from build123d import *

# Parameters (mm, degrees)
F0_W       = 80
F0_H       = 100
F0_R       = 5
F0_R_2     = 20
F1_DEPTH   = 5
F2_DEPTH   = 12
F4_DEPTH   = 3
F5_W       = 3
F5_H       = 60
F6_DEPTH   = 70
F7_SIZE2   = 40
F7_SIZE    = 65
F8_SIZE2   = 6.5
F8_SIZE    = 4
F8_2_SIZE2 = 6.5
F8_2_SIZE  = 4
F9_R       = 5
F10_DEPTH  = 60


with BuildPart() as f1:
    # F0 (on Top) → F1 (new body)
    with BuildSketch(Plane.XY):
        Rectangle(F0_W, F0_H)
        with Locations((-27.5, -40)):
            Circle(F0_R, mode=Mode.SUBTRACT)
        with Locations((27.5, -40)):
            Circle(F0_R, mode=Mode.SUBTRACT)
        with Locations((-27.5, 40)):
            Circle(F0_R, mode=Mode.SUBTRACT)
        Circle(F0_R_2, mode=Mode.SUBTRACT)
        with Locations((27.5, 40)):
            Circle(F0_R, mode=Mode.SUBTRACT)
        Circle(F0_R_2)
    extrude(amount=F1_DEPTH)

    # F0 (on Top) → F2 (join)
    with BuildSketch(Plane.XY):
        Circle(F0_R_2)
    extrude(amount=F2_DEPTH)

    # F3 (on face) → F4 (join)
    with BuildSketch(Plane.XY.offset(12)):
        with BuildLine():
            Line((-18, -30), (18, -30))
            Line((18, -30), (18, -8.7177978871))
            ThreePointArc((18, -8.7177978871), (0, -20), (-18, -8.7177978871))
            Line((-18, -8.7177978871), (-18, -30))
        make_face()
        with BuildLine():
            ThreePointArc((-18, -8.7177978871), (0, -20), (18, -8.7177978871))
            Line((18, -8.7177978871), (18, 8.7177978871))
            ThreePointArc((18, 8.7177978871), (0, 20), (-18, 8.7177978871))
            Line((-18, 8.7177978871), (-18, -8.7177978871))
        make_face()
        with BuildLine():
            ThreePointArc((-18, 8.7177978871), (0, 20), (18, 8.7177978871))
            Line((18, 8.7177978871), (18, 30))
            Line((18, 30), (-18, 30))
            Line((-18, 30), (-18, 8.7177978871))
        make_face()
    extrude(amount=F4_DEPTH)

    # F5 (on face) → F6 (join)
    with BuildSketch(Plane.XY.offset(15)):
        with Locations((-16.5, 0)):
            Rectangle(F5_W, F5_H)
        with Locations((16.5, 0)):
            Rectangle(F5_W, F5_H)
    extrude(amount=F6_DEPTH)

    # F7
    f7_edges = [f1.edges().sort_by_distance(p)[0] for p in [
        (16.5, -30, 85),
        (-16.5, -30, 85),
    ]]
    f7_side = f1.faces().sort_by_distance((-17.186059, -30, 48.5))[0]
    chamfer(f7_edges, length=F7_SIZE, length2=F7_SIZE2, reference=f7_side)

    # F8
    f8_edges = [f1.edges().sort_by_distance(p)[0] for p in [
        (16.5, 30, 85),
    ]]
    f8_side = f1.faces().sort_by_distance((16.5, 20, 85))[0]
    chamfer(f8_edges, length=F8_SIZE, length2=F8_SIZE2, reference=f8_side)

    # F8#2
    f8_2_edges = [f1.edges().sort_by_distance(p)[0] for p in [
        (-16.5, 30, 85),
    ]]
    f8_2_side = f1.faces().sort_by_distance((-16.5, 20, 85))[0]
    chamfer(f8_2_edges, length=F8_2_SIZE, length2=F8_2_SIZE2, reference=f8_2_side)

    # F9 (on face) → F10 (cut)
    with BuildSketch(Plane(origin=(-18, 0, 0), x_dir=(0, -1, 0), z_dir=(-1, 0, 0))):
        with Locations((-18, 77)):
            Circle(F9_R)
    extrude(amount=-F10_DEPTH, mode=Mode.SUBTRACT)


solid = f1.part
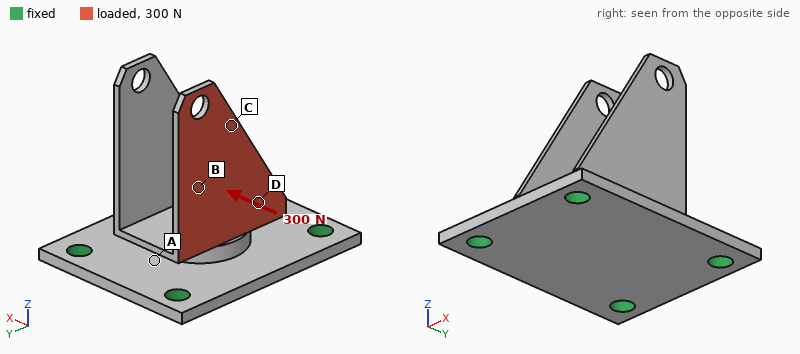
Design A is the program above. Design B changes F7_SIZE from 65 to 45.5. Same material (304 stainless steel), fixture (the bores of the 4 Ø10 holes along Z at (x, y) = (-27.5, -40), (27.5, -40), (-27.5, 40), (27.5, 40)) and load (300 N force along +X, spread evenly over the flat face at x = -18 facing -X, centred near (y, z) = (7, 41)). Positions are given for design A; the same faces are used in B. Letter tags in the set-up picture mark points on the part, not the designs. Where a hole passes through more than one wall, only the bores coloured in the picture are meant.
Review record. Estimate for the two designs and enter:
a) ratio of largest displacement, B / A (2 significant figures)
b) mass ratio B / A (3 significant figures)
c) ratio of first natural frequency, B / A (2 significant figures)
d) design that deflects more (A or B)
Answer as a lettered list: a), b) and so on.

a) 0.92
b) 1.03
c) 0.98
d) A
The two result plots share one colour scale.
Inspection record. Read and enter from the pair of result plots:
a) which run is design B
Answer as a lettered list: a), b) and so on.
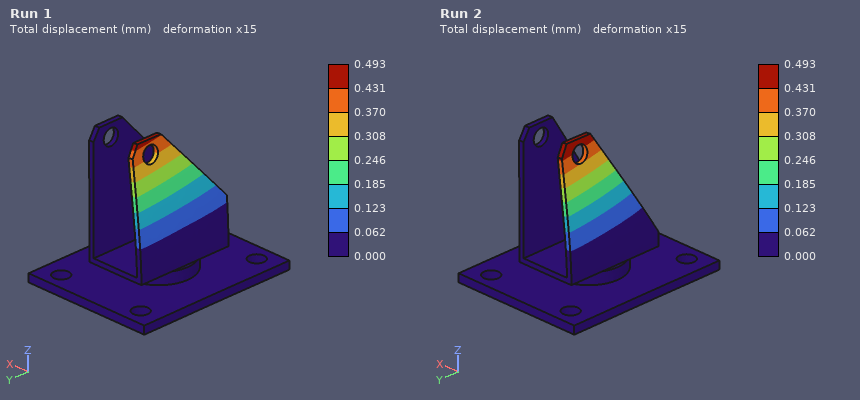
a) Run 1
